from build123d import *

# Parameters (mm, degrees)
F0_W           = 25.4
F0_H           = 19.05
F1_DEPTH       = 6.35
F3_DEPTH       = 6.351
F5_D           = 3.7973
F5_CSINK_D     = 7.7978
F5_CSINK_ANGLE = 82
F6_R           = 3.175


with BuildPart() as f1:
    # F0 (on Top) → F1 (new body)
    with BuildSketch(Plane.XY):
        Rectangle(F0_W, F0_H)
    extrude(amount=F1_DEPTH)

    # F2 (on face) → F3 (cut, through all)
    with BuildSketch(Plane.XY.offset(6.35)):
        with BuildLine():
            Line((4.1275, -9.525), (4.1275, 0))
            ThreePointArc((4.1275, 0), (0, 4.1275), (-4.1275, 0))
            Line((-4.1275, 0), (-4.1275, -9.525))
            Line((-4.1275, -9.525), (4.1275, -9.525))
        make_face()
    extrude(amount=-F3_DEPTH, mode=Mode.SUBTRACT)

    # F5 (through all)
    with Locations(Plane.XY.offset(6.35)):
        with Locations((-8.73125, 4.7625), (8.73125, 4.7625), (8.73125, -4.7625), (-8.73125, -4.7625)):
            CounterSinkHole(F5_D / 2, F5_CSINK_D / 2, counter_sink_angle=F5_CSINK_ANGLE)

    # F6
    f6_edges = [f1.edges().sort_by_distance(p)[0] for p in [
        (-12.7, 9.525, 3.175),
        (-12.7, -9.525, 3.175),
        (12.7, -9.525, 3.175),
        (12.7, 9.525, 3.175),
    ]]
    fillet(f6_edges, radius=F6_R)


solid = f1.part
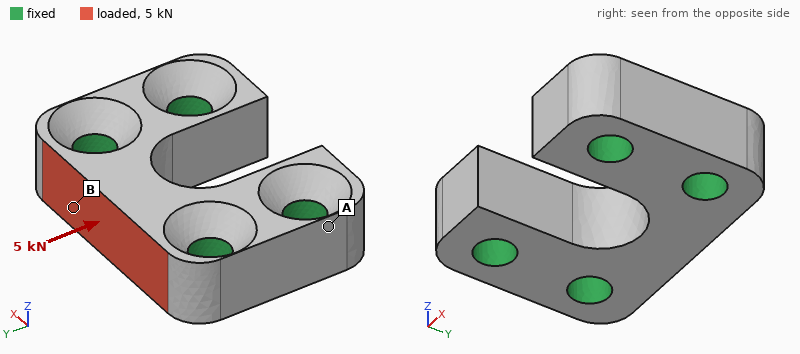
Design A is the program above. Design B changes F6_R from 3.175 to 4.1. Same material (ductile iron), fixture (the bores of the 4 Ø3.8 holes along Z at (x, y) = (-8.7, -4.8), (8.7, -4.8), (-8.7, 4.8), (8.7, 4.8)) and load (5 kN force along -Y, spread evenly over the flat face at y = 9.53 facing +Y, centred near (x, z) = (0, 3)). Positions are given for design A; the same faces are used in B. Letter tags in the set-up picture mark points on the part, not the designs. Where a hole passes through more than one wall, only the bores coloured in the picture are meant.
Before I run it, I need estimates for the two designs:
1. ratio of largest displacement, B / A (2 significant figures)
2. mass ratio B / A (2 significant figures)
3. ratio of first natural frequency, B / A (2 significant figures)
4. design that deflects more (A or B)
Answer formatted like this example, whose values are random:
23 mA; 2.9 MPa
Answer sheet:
1.1; 0.98; 1.0; B
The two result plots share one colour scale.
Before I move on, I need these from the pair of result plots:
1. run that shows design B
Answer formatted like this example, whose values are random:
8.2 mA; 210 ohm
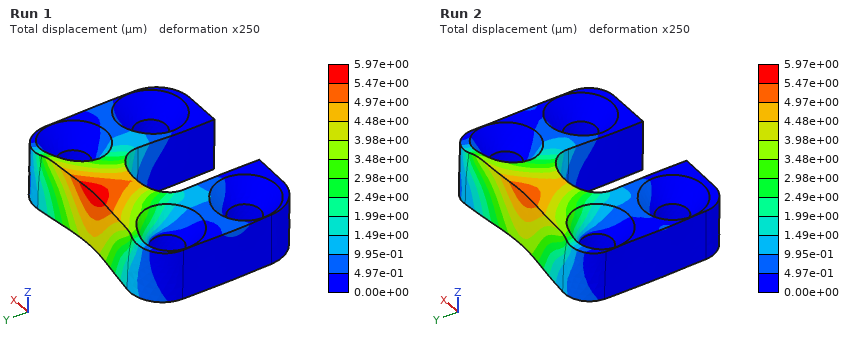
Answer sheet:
Run 1
